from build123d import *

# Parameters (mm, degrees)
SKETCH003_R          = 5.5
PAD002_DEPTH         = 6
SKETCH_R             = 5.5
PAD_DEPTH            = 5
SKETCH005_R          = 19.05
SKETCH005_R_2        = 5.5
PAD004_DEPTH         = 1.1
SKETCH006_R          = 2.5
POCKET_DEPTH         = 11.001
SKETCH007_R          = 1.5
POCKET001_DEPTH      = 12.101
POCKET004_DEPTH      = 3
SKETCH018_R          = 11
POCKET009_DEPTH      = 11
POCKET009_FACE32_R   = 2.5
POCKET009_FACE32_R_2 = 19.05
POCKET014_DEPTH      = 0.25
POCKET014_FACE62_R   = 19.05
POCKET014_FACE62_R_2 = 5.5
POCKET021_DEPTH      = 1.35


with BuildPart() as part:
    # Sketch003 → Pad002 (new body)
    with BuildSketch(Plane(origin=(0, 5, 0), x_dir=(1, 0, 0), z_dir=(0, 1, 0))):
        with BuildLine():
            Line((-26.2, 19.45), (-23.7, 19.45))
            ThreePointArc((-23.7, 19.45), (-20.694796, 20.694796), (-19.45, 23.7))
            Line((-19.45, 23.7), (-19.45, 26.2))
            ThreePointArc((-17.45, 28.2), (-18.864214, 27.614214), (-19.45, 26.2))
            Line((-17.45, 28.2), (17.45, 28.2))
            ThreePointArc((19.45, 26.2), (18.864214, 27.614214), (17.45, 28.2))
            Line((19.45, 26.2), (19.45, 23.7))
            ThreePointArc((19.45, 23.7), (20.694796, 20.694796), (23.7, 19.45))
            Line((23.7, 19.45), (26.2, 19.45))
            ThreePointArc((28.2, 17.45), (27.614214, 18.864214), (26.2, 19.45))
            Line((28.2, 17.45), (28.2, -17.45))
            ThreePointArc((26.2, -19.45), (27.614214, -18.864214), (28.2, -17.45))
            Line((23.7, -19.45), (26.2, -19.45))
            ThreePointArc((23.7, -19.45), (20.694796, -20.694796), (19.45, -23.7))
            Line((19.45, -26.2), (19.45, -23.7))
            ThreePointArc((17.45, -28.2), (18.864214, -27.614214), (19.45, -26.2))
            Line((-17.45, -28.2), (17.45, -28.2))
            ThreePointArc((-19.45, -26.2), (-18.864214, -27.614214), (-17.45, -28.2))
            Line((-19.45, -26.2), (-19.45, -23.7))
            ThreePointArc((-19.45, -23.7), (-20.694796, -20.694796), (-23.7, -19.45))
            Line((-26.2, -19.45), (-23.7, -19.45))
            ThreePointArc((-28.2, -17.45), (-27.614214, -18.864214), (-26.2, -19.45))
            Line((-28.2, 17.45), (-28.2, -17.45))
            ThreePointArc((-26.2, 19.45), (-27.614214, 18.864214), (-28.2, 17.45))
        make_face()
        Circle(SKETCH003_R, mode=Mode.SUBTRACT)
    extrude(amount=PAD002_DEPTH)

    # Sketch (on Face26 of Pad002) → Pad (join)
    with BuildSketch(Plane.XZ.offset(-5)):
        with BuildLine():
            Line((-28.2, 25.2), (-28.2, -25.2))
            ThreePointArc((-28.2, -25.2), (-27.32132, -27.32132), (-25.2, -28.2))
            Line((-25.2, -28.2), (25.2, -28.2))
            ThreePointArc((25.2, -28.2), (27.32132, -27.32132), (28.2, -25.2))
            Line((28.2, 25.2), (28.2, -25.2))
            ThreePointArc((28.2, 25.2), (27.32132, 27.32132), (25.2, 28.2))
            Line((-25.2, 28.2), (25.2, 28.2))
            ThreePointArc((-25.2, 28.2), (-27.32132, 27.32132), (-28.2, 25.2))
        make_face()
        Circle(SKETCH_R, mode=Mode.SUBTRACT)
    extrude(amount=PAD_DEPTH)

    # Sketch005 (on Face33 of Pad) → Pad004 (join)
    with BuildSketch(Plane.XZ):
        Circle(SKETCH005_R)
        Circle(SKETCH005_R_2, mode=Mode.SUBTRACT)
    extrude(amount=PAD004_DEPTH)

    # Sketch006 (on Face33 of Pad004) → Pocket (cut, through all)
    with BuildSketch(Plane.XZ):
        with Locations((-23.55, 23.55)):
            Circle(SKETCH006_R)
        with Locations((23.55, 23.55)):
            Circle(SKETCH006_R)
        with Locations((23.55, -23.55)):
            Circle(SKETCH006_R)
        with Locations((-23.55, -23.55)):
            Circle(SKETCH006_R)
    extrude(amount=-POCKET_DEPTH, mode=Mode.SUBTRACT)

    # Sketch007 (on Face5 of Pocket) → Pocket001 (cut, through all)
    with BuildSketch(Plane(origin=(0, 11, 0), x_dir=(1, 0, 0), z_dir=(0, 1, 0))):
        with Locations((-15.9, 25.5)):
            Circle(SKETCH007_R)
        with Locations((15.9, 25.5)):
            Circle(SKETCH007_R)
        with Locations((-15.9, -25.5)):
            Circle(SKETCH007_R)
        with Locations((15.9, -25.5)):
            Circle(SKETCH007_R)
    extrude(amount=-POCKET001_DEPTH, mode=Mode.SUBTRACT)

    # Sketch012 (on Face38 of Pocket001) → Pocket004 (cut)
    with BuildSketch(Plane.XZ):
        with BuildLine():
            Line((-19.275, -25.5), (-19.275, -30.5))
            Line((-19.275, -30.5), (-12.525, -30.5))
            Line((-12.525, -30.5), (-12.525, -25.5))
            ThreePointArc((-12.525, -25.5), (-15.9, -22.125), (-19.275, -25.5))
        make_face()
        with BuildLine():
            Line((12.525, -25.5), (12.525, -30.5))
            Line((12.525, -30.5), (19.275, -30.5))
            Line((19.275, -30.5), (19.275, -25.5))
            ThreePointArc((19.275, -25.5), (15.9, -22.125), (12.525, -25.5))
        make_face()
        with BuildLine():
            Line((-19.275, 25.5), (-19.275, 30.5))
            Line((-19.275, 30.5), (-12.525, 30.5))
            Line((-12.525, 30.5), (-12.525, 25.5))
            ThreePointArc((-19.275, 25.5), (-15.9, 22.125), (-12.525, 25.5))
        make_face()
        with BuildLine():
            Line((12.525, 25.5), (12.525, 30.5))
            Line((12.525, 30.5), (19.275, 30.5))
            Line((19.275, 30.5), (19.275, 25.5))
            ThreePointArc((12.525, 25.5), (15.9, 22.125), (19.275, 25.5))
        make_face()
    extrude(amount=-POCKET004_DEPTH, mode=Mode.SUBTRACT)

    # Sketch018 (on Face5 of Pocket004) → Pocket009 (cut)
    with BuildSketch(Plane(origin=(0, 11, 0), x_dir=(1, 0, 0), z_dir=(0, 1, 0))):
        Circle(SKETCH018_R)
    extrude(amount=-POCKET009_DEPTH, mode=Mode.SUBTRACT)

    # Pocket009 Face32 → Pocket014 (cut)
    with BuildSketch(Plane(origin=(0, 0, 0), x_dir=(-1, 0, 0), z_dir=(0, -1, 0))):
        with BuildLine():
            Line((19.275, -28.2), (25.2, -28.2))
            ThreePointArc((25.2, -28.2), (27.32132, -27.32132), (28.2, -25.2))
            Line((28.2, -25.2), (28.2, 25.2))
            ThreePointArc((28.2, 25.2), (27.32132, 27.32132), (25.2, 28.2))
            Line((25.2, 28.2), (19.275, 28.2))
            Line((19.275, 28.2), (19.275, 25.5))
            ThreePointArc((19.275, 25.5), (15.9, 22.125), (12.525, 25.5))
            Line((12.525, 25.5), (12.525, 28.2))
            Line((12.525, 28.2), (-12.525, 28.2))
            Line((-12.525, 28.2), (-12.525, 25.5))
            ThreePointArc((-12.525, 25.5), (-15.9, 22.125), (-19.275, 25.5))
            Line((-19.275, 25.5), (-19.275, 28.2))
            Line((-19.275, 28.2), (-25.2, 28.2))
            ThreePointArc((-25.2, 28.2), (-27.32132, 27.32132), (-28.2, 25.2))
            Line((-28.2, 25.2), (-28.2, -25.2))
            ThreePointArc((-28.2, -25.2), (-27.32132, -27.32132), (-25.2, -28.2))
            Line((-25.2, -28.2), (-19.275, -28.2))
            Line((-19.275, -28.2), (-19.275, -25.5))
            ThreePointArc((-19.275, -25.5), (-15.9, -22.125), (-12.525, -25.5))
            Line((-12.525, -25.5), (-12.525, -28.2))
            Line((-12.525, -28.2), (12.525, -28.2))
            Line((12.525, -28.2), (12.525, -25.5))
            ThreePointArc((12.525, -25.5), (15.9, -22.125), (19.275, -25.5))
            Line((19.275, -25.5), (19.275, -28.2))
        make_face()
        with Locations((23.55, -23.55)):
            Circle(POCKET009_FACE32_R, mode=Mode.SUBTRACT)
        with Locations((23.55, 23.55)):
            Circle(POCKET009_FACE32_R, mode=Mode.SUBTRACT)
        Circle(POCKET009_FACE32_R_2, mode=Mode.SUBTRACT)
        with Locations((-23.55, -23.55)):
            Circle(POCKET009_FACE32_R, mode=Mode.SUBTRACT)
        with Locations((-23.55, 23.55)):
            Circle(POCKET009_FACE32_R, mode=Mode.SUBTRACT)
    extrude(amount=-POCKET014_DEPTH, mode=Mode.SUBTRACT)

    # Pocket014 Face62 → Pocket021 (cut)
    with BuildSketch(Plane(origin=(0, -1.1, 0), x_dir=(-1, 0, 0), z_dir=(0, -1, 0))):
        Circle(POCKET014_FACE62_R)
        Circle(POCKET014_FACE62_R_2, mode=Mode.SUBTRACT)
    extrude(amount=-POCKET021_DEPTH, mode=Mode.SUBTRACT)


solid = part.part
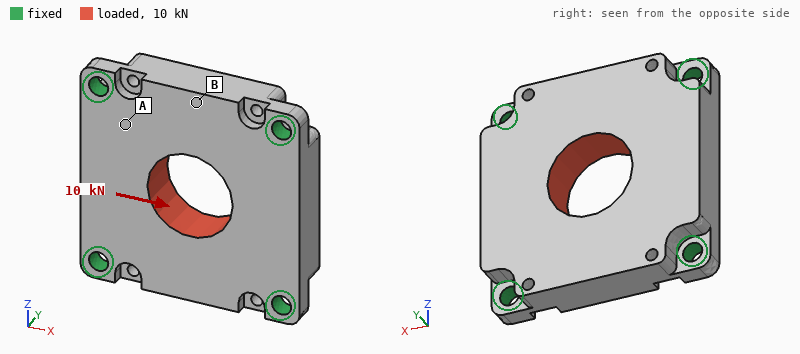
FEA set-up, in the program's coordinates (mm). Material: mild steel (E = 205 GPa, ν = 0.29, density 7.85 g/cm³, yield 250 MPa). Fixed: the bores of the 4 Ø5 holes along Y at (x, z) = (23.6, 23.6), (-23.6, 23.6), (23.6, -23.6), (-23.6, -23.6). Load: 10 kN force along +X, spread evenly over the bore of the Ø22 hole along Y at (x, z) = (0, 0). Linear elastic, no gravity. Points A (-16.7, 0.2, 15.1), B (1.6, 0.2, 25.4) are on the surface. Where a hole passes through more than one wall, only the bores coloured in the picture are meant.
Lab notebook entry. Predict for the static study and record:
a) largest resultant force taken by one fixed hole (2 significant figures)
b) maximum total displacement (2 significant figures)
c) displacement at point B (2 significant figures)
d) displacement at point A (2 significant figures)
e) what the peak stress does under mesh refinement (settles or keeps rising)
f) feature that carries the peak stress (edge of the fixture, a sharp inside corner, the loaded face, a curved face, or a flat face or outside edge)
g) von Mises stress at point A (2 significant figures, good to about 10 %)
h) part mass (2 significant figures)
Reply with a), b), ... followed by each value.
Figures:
a) 2.7 kN
b) 4.9 µm
c) 2.7 µm
d) 2.6 µm
e) keeps rising
f) edge of the fixture
g) 27 MPa
h) 210 g
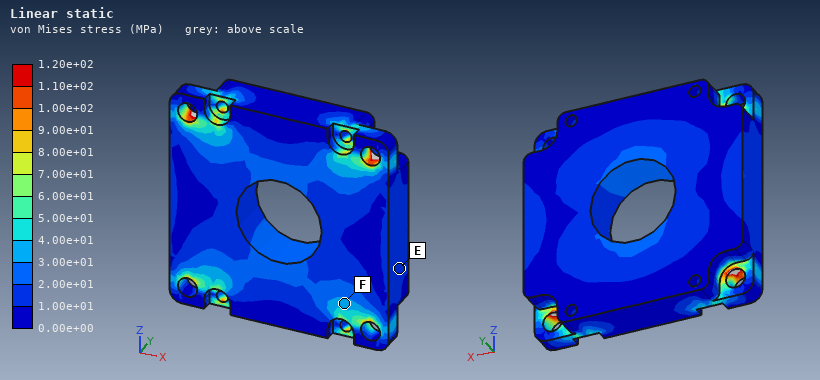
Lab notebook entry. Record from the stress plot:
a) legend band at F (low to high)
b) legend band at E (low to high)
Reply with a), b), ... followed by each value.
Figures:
a) 3.00e+01 to 4.00e+01 MPa
b) 1.00e+01 to 2.00e+01 MPa
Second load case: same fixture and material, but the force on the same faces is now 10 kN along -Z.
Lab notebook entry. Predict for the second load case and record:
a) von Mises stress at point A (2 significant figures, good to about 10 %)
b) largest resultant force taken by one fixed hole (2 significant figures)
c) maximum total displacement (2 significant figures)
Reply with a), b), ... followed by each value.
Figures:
a) 28 MPa
b) 2.7 kN
c) 4.4 µm
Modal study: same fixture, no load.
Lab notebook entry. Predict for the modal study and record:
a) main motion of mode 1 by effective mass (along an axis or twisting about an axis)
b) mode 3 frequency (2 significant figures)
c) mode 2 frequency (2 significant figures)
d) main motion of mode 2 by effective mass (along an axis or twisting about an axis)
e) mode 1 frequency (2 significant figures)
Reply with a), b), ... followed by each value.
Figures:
a) along Y
b) 17 kHz
c) 16 kHz
d) twisting about X
e) 11 kHz
